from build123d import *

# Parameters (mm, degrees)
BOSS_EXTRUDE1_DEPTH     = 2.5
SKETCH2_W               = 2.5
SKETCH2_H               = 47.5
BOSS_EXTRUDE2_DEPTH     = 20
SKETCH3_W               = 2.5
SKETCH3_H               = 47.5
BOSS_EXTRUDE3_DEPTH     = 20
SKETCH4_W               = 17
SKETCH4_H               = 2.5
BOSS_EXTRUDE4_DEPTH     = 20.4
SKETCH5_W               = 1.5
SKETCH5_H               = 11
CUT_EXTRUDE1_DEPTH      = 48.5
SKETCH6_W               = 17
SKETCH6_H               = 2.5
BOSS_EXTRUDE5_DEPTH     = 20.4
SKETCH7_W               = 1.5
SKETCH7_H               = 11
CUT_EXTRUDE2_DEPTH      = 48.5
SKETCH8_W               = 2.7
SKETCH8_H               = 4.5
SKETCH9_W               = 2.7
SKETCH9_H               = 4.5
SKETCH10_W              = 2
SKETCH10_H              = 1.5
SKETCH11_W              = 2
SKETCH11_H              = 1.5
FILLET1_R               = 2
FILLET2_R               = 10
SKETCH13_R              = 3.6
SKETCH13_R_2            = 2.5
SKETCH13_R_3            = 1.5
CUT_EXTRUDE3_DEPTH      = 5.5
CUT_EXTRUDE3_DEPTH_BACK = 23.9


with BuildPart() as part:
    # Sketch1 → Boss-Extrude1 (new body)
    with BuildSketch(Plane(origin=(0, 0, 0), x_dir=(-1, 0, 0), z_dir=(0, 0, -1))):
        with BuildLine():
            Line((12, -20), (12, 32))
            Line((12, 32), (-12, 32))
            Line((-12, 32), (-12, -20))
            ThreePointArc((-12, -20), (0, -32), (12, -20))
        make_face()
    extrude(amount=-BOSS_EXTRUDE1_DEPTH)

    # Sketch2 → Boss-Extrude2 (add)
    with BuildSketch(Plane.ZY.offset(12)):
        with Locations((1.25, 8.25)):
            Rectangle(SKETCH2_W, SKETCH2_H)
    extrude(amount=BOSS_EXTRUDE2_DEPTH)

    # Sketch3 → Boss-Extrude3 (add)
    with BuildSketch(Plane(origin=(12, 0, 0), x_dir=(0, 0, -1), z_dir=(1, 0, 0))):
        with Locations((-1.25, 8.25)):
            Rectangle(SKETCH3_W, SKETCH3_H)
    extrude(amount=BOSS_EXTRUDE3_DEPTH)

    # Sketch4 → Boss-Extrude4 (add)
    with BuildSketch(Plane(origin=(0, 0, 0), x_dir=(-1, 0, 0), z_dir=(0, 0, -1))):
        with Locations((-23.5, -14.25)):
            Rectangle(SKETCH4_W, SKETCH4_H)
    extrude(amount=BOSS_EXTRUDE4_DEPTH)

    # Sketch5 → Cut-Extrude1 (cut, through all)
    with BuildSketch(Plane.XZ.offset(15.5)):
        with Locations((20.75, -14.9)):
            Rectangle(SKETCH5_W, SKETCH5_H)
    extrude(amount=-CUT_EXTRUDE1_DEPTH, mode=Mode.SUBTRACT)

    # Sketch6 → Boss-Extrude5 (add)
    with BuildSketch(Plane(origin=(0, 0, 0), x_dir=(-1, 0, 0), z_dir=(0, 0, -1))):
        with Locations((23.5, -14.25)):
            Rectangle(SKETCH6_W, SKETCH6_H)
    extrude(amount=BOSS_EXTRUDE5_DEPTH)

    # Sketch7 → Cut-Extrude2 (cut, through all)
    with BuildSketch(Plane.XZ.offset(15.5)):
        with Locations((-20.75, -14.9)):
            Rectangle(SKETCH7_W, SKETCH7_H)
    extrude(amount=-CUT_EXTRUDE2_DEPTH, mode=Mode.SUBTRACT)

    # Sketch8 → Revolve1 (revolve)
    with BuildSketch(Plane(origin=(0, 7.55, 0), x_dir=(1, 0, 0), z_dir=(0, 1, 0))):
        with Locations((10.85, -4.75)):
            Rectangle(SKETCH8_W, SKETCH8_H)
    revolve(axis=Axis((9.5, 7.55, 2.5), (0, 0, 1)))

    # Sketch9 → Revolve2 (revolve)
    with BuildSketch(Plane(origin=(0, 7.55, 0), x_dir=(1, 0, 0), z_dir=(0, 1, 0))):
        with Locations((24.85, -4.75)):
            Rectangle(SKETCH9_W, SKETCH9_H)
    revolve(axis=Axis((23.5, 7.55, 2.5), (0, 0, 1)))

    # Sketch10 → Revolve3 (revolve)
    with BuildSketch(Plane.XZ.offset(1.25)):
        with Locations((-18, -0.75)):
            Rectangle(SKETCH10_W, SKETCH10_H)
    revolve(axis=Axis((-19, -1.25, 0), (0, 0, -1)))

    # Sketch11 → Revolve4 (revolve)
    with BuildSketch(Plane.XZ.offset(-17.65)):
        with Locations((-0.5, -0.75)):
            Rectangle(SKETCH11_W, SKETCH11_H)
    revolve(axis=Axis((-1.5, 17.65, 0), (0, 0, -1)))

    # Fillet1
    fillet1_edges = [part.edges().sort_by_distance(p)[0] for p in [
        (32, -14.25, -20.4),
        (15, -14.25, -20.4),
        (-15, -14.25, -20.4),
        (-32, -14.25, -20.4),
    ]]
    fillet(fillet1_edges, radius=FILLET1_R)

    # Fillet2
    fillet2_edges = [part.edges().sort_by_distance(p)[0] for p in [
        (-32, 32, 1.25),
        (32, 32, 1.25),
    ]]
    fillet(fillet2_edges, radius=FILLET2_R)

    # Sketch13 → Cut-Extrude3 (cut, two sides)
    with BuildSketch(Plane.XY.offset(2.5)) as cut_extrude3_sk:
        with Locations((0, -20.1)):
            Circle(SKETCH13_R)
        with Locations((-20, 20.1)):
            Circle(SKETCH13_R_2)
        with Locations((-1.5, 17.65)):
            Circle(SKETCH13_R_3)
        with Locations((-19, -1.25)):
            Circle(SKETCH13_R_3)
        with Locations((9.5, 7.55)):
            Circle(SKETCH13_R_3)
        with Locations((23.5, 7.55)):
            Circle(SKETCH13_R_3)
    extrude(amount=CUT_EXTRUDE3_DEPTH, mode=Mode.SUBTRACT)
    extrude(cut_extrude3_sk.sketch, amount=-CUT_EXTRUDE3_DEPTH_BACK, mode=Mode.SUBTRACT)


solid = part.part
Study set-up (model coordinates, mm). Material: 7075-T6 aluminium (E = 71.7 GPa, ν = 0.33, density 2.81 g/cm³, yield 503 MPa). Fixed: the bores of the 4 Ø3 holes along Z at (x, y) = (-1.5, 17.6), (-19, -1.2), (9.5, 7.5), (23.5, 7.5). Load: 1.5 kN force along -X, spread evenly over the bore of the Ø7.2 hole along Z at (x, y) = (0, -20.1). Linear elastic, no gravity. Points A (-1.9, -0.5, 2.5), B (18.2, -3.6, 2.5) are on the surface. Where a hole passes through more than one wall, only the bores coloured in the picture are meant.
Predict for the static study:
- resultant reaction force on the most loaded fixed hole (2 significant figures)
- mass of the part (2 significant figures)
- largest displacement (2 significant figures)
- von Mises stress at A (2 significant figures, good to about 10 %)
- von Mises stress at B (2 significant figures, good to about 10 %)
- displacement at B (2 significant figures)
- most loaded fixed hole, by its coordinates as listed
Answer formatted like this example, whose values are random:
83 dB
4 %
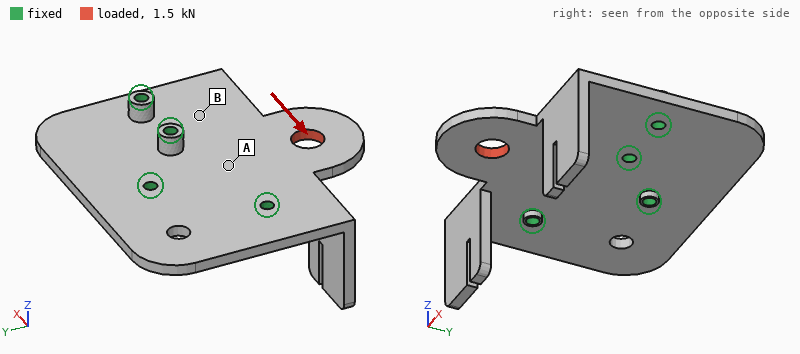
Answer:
1.2 kN
28 g
28 µm
9.2 MPa
23 MPa
5.1 µm
(-19, -1.2)
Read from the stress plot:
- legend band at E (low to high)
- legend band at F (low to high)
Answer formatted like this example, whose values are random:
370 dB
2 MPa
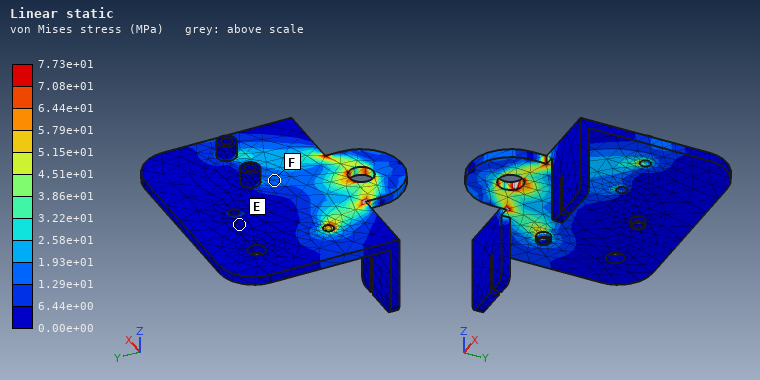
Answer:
0.00e+00 to 6.44e+00 MPa
1.29e+01 to 1.93e+01 MPa
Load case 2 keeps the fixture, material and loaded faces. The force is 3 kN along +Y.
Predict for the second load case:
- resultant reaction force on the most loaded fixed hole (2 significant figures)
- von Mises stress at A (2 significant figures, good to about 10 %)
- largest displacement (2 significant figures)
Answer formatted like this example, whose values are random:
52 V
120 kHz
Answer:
1.0 kN
29 MPa
23 µm
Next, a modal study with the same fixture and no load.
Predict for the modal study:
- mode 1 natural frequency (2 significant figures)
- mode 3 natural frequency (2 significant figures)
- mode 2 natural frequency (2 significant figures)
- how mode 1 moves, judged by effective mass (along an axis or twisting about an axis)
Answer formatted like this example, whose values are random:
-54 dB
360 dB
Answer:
1900 Hz
2900 Hz
2500 Hz
along Z
